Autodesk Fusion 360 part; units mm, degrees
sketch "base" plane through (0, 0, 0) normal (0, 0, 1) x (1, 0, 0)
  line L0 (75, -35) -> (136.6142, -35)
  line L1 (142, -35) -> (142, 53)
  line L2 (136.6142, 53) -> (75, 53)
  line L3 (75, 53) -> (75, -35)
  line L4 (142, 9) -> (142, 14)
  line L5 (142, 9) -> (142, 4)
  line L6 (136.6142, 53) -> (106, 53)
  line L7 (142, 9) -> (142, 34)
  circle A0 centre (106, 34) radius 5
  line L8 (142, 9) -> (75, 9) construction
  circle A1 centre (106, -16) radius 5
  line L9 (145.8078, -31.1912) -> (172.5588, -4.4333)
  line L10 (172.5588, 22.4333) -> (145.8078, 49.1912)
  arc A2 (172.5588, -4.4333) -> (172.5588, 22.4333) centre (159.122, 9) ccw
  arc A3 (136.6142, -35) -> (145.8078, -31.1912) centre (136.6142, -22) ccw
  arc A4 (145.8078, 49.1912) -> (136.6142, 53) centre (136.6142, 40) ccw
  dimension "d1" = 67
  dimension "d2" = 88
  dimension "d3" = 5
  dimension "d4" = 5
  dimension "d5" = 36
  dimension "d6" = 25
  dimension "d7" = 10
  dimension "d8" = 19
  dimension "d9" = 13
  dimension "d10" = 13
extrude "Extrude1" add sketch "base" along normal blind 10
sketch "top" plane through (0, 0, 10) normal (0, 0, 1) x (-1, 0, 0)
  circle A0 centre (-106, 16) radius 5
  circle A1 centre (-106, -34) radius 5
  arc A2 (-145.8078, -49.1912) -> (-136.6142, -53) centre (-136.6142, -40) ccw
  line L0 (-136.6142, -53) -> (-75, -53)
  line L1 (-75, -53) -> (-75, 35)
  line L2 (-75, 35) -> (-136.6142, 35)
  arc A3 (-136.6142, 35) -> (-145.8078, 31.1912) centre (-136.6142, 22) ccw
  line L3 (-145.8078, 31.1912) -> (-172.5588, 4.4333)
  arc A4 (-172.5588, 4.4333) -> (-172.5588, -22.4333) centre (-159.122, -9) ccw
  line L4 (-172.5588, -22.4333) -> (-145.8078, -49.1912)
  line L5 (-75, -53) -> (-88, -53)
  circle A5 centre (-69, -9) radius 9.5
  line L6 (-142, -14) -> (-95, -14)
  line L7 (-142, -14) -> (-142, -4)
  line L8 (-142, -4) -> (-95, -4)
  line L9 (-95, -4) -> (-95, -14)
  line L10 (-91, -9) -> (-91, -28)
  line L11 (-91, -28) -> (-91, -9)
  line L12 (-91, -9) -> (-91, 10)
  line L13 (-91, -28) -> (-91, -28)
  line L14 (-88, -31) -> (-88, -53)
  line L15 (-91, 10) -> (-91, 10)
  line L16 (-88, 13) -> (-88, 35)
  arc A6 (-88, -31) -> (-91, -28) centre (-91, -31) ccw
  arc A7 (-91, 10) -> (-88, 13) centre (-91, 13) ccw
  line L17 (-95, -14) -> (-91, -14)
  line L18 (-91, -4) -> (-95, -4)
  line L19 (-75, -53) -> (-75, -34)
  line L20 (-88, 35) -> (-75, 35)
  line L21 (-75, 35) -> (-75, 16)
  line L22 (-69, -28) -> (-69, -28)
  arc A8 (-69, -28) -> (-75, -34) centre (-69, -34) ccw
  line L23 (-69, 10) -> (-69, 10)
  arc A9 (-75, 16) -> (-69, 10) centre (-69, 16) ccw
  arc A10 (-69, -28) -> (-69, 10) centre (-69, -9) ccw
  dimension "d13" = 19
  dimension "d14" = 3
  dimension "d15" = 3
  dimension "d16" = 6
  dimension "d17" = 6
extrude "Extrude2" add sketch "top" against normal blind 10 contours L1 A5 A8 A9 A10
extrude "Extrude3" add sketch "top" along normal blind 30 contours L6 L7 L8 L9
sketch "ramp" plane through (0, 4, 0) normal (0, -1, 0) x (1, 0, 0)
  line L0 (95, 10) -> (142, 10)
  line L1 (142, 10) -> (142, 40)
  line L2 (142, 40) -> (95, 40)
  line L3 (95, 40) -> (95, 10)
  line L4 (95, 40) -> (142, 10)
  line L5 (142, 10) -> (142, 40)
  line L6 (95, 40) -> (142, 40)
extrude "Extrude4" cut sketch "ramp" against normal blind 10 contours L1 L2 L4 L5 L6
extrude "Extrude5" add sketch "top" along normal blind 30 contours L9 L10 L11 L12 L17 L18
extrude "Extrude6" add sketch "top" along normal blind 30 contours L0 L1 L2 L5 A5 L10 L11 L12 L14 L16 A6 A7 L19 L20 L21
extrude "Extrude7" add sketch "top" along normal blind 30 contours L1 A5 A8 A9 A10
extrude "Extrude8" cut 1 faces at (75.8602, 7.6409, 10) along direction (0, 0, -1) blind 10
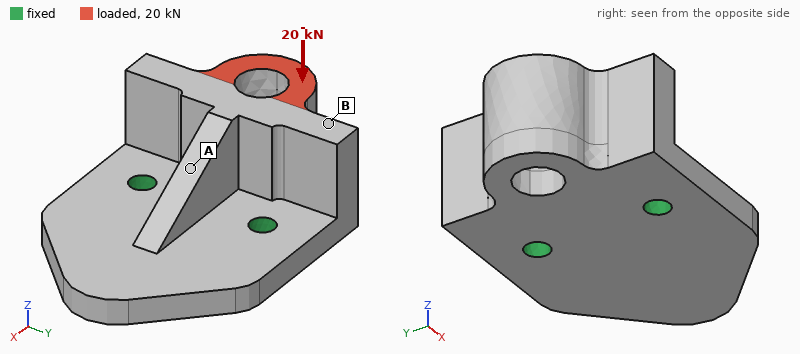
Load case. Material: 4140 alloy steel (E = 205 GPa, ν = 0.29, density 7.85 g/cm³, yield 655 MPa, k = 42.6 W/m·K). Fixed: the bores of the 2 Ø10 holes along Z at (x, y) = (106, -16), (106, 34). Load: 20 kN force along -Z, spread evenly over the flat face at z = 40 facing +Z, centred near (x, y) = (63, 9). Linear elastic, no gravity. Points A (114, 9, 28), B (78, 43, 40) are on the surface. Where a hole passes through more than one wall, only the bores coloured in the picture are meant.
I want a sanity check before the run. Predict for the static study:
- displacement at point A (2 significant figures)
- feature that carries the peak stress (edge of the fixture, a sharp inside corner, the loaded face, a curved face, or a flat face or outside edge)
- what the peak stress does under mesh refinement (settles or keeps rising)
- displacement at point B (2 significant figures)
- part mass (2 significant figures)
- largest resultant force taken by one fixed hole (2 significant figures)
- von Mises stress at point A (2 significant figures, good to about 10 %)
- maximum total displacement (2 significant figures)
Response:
0.088 mm
edge of the fixture
keeps rising
0.19 mm
1.1 kg
11 kN
140 MPa
0.29 mm
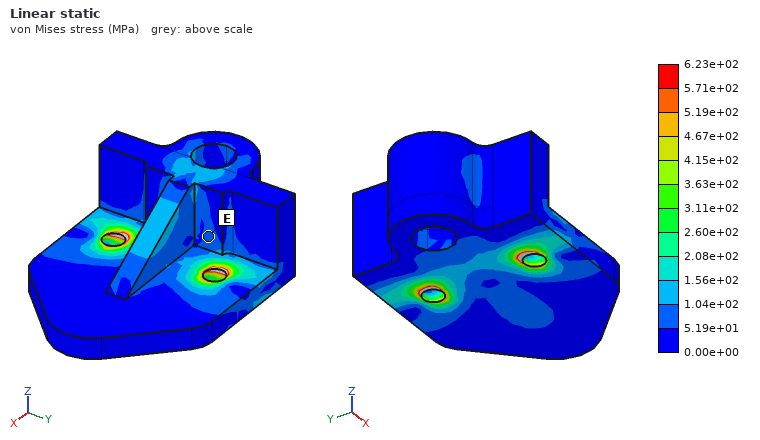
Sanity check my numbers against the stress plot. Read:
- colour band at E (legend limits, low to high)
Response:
5.19e+01 to 1.04e+02 MPa
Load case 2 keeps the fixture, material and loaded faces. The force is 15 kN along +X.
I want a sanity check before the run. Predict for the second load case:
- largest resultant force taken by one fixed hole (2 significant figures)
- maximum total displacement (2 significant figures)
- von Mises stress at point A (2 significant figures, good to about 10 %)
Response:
7.6 kN
0.21 mm
110 MPa
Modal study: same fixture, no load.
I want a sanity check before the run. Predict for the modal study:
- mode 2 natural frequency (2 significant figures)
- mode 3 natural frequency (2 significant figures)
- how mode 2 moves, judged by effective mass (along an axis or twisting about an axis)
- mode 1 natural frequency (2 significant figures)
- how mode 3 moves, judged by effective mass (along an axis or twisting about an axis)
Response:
3700 Hz
5500 Hz
along Z
2100 Hz
along Y
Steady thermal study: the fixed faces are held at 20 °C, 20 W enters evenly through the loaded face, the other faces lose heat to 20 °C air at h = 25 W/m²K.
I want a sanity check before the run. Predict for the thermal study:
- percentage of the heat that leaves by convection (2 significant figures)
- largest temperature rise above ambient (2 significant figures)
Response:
27 %
30 K
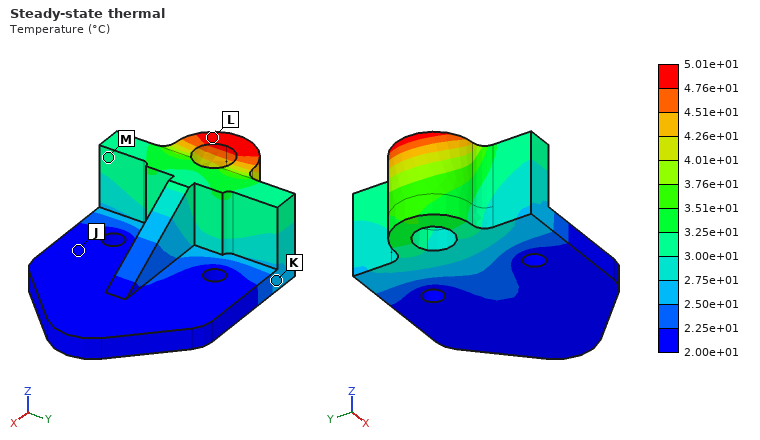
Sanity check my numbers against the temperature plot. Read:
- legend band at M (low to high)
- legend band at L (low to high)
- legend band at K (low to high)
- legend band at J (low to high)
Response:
3.00e+01 to 3.25e+01 °C
4.76e+01 to 5.01e+01 °C
2.50e+01 to 2.75e+01 °C
2.00e+01 to 2.25e+01 °C
